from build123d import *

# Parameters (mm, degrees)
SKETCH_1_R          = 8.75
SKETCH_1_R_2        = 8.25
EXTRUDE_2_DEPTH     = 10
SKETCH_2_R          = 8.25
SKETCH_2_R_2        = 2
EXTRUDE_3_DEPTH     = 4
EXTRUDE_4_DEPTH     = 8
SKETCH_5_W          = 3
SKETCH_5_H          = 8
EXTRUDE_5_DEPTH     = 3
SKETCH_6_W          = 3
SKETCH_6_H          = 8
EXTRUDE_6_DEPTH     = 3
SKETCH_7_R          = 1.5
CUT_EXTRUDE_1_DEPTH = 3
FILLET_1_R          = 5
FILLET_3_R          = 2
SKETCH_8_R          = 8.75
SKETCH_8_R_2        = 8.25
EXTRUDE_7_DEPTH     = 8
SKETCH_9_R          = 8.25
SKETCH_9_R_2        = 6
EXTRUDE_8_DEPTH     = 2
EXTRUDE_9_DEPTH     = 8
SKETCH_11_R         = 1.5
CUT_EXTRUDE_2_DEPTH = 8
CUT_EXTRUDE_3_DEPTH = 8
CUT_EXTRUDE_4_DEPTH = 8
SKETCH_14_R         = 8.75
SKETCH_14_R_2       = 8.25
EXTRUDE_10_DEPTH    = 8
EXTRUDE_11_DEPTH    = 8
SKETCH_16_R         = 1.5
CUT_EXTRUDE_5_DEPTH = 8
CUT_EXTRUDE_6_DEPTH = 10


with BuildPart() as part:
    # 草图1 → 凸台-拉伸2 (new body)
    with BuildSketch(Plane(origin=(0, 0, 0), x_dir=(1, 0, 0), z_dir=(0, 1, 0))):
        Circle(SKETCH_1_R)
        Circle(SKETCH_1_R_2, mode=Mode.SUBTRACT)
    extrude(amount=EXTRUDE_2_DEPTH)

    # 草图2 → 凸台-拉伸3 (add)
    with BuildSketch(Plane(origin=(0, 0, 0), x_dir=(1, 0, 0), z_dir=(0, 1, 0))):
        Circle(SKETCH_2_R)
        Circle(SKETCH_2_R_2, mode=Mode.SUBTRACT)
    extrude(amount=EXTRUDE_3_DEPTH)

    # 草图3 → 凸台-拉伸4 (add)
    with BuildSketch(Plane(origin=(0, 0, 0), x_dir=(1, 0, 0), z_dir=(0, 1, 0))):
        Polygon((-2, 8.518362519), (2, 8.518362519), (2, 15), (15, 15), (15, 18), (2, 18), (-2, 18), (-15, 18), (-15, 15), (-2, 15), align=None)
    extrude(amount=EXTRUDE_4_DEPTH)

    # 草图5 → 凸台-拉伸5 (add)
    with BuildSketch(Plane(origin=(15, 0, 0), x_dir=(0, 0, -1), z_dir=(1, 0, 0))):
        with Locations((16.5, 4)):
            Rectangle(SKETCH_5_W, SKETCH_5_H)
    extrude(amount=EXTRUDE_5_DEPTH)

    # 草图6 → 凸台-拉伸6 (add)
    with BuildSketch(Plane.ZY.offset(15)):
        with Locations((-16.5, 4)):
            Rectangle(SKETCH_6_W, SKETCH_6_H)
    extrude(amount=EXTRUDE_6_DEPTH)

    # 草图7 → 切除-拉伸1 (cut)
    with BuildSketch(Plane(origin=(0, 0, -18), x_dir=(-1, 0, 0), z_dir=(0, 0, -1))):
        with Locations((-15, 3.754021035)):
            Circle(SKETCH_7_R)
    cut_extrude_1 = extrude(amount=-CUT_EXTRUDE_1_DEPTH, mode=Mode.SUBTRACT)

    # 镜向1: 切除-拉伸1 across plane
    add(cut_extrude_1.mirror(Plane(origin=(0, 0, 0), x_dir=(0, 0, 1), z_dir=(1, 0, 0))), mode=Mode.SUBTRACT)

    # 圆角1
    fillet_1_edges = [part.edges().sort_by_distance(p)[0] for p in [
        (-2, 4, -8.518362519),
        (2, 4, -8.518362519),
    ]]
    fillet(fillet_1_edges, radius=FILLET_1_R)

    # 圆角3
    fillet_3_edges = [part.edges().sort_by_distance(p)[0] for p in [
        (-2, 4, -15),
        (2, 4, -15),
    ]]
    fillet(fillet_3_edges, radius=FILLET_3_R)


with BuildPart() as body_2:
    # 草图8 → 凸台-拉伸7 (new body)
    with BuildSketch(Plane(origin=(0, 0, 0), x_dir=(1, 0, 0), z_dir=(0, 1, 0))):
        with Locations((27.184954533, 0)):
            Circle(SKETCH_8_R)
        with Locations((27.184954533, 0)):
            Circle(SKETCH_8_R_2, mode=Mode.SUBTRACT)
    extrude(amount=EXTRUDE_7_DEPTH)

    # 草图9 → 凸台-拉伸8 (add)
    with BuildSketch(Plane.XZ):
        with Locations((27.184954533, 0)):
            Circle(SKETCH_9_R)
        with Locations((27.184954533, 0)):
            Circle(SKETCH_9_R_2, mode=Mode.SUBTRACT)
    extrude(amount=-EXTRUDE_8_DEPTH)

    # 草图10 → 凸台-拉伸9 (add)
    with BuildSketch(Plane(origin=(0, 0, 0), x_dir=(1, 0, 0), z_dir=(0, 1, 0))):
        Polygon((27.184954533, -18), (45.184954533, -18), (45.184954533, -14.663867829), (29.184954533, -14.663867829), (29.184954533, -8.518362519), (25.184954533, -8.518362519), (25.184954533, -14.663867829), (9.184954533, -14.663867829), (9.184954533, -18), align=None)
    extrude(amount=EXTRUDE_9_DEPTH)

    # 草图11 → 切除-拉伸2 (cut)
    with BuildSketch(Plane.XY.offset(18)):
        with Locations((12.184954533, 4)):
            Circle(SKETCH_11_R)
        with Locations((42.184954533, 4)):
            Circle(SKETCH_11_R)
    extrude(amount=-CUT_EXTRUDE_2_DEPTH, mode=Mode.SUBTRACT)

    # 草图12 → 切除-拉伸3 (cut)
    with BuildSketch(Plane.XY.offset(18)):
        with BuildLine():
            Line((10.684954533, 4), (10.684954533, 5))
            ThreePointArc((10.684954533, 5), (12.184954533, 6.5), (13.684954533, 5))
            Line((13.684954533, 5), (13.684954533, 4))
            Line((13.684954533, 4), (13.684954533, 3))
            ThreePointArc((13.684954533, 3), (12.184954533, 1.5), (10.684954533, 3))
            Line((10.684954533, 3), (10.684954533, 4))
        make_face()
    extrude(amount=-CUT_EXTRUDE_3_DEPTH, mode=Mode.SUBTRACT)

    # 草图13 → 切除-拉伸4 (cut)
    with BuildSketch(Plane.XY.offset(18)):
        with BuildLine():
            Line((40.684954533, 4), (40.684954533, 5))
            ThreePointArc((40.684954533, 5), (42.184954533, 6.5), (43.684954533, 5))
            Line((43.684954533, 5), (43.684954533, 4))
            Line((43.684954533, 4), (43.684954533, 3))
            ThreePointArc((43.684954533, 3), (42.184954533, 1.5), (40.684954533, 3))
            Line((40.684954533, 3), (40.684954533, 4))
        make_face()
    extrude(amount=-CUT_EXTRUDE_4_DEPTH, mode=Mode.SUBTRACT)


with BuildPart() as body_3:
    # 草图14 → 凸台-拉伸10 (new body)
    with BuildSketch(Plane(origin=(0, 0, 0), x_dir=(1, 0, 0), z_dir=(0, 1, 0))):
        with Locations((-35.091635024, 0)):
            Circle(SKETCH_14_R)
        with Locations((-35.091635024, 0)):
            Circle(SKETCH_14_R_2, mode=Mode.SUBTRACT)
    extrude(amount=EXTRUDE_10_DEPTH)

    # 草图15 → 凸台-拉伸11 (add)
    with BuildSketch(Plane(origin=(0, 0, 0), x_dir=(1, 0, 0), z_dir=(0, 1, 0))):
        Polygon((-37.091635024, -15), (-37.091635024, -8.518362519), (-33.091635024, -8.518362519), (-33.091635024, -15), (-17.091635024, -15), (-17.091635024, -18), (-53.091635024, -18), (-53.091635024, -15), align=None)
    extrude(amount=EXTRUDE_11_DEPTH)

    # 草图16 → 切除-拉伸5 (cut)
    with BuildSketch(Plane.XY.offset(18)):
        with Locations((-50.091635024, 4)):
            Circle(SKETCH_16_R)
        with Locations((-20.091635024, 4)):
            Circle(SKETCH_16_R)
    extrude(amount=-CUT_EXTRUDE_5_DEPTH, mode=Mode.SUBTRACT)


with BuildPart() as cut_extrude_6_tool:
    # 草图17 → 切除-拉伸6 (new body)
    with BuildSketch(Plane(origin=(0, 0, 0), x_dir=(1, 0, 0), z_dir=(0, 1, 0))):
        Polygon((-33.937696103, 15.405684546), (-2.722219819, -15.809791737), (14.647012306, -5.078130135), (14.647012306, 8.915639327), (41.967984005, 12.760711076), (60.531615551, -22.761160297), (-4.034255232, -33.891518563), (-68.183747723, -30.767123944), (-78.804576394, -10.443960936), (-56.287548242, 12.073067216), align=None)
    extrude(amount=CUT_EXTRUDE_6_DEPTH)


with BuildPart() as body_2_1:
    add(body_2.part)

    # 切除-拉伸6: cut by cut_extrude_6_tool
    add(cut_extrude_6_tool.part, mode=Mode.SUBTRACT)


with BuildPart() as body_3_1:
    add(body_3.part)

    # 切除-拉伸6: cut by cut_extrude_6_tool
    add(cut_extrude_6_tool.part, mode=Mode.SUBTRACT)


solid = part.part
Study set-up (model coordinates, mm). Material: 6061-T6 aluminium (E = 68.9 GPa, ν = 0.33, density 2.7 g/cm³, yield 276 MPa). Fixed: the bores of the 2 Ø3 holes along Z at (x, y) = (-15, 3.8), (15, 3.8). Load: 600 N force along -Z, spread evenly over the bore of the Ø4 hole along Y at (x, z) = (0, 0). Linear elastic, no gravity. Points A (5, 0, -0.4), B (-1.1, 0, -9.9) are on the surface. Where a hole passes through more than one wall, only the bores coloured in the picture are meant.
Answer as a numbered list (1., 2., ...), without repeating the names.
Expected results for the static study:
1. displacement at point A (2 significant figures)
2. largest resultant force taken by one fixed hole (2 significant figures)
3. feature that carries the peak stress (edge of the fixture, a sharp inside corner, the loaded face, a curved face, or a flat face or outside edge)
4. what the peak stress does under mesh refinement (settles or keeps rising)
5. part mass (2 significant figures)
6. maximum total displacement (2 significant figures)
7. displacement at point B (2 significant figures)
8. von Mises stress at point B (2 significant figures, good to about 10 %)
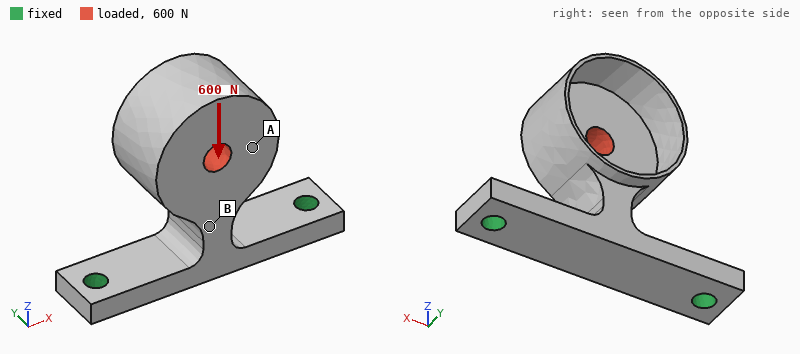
1. 0.10 mm
2. 320 N
3. edge of the fixture
4. keeps rising
5. 5.8 g
6. 0.14 mm
7. 0.073 mm
8. 36 MPa
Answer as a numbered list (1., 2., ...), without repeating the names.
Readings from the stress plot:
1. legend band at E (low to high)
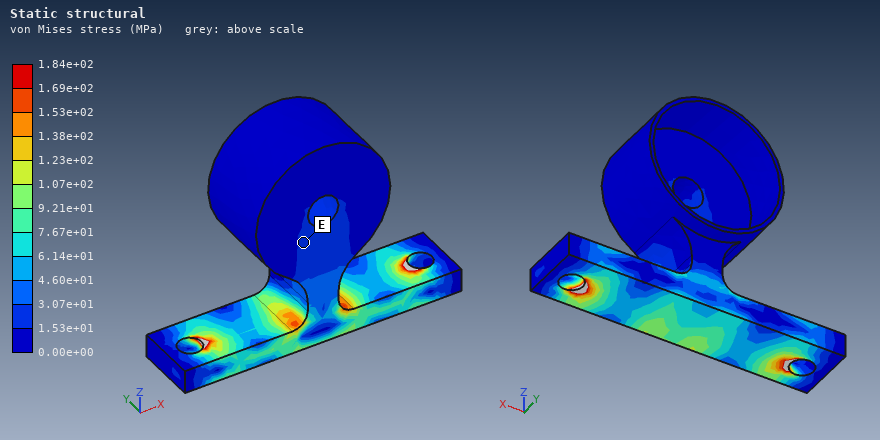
1. 1.53e+01 to 3.07e+01 MPa
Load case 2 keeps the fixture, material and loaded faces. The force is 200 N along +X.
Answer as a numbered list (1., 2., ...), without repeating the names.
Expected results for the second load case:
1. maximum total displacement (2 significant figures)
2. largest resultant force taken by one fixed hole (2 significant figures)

1. 0.20 mm
2. 200 N
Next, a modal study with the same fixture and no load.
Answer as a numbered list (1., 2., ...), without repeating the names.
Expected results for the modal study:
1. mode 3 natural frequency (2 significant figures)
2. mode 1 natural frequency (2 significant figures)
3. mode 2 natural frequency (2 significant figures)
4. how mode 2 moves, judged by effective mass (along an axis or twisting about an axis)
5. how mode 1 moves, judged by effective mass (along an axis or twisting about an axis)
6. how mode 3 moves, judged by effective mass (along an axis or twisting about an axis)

1. 8500 Hz
2. 2500 Hz
3. 3400 Hz
4. along X
5. along Y
6. along Z
